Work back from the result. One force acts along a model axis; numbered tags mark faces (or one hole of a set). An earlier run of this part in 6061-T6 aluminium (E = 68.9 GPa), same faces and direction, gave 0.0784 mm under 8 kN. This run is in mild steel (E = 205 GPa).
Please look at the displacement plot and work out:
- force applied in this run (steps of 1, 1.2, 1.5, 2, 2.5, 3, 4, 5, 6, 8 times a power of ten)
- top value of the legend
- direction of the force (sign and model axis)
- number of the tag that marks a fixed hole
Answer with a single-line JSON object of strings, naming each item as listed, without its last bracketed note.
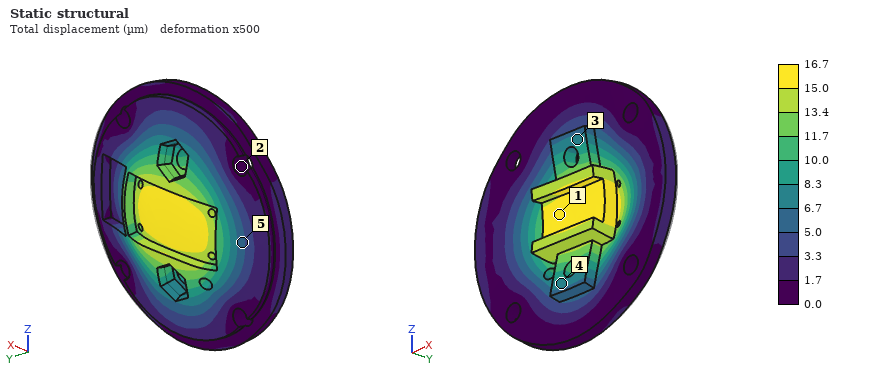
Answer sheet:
{"force applied in this run": "5 kN", "top value of the legend": "16.7 µm", "direction of the force": "+Y", "number of the tag that marks a fixed hole": "2"}
